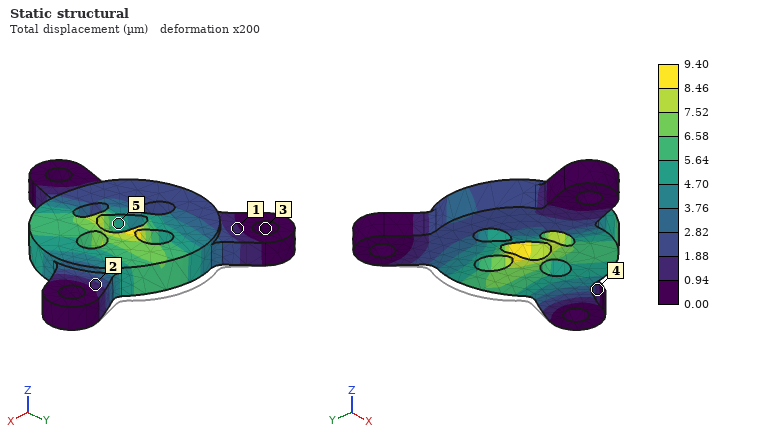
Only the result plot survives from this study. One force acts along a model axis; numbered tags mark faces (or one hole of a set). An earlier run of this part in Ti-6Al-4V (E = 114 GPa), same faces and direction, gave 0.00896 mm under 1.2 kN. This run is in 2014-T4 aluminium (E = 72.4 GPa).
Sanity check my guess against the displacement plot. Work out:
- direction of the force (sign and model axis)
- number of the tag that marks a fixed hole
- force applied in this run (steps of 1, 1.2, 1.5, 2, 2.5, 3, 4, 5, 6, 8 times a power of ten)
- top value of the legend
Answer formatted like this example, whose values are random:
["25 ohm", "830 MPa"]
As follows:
["-Y", "3", "800 N", "9.40 µm"]
